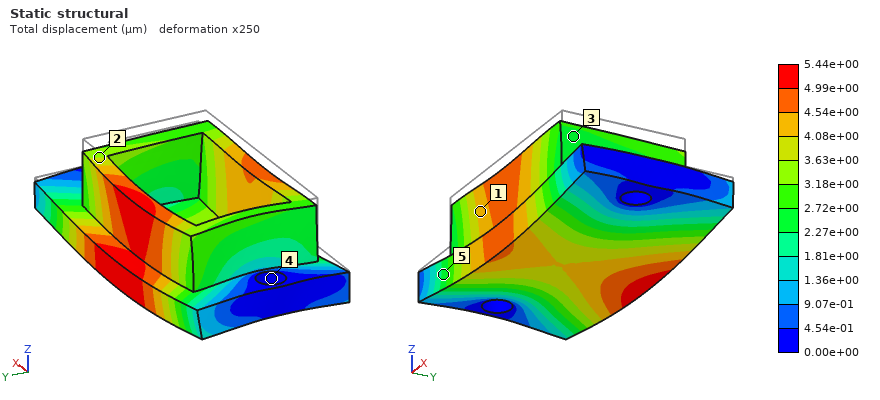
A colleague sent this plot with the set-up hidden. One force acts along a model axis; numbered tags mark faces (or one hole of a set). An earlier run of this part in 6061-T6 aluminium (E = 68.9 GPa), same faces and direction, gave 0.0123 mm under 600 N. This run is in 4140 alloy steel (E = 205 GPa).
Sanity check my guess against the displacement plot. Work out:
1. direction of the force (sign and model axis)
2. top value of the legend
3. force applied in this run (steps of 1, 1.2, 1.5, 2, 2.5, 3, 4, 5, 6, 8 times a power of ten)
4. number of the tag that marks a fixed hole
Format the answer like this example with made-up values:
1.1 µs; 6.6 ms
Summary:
-Z; 5.44e+00 µm; 800 N; 4
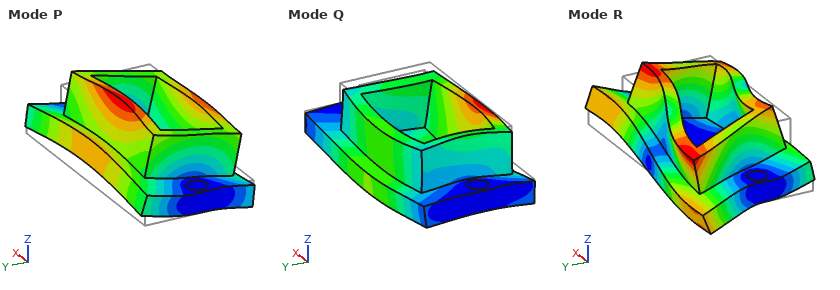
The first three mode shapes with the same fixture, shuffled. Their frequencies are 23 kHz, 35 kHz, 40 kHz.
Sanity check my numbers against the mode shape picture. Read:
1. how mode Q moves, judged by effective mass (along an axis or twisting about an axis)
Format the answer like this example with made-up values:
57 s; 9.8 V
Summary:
along Z
